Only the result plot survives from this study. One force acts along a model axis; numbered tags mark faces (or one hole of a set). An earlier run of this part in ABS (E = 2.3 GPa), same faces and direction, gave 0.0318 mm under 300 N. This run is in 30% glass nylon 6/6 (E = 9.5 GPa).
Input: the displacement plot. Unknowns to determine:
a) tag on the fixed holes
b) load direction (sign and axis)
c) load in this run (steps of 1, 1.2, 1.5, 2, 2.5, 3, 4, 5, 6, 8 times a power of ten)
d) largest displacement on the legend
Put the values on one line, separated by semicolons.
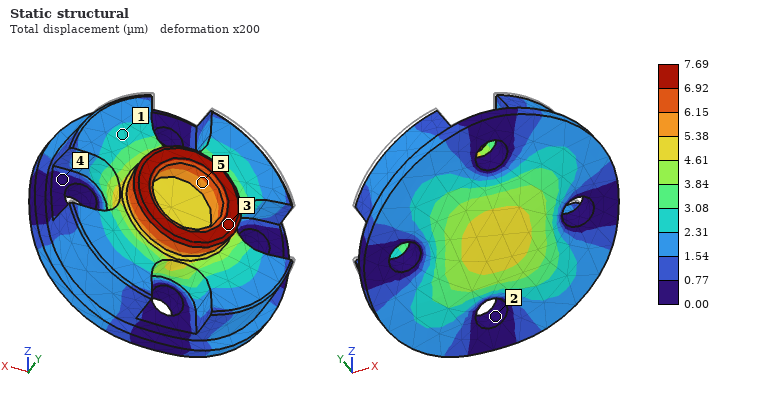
2; -Y; 300 N; 7.69 µm
